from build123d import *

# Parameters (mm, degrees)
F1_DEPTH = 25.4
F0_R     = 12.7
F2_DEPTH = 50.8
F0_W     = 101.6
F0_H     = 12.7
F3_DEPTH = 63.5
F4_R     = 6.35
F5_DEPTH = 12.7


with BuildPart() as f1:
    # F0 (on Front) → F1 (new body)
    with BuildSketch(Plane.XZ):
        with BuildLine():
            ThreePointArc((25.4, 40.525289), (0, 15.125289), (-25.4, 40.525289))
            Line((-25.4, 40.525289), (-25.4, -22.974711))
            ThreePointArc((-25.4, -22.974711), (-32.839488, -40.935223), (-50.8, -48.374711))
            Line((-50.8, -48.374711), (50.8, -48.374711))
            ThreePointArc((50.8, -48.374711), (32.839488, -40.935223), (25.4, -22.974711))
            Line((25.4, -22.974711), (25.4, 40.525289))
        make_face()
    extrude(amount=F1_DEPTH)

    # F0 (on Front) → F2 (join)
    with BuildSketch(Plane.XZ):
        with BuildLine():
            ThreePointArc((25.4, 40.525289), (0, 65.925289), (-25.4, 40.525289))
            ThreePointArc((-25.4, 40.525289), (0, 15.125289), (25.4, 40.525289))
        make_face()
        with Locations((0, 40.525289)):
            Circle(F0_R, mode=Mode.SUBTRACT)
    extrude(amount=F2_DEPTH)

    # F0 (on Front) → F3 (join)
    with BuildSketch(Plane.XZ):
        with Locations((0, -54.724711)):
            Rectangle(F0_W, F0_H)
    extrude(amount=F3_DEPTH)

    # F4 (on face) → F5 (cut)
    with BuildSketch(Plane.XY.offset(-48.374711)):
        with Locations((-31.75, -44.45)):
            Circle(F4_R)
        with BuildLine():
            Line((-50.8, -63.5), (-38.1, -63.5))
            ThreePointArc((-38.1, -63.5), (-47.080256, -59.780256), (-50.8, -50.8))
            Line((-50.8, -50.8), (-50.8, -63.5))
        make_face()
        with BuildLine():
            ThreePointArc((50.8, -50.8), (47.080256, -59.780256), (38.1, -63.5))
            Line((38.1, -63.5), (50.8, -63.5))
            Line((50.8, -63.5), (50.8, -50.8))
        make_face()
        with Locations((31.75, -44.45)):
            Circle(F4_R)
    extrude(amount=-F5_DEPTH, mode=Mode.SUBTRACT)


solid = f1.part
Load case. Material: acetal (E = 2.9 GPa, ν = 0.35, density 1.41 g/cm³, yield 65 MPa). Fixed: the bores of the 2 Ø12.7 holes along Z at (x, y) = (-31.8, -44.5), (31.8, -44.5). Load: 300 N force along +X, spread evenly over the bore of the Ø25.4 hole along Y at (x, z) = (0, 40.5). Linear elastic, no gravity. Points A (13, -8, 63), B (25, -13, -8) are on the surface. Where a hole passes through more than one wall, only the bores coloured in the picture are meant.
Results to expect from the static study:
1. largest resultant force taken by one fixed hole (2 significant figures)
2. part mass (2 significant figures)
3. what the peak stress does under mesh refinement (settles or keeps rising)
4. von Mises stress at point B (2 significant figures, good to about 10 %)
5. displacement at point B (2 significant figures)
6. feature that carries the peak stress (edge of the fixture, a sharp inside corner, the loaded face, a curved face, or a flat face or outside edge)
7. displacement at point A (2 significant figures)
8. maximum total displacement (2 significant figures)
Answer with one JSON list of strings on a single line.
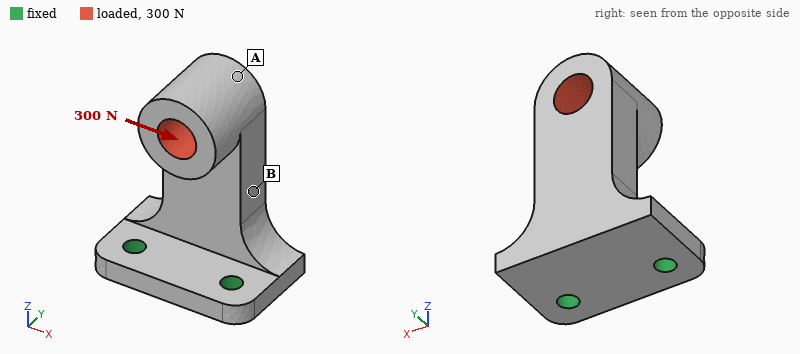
["460 N", "350 g", "keeps rising", "1.5 MPa", "0.15 mm", "edge of the fixture", "0.36 mm", "0.46 mm"]
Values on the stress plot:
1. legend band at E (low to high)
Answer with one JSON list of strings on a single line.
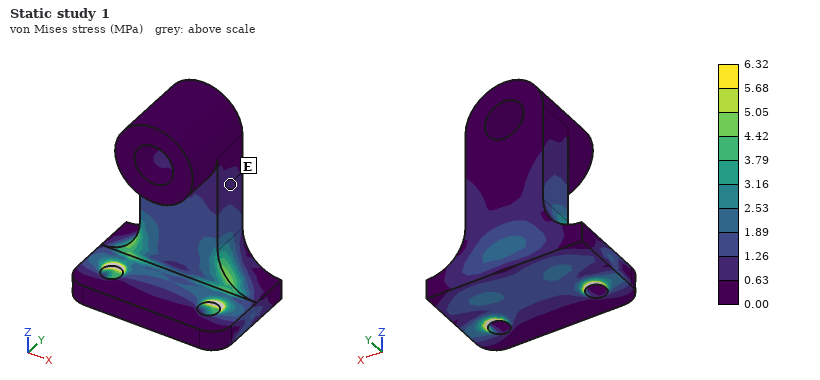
["0.63 to 1.26 MPa"]
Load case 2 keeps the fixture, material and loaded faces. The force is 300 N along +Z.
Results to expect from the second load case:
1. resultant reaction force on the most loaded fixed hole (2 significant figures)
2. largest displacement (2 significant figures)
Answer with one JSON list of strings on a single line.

["150 N", "68 µm"]
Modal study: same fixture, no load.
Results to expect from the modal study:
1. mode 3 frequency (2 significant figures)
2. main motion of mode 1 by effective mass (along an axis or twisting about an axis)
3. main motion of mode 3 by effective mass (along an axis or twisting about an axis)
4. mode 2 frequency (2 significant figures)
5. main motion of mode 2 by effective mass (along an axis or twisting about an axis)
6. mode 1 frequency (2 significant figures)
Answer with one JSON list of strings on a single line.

["850 Hz", "along Y", "along Z", "410 Hz", "along X", "180 Hz"]
